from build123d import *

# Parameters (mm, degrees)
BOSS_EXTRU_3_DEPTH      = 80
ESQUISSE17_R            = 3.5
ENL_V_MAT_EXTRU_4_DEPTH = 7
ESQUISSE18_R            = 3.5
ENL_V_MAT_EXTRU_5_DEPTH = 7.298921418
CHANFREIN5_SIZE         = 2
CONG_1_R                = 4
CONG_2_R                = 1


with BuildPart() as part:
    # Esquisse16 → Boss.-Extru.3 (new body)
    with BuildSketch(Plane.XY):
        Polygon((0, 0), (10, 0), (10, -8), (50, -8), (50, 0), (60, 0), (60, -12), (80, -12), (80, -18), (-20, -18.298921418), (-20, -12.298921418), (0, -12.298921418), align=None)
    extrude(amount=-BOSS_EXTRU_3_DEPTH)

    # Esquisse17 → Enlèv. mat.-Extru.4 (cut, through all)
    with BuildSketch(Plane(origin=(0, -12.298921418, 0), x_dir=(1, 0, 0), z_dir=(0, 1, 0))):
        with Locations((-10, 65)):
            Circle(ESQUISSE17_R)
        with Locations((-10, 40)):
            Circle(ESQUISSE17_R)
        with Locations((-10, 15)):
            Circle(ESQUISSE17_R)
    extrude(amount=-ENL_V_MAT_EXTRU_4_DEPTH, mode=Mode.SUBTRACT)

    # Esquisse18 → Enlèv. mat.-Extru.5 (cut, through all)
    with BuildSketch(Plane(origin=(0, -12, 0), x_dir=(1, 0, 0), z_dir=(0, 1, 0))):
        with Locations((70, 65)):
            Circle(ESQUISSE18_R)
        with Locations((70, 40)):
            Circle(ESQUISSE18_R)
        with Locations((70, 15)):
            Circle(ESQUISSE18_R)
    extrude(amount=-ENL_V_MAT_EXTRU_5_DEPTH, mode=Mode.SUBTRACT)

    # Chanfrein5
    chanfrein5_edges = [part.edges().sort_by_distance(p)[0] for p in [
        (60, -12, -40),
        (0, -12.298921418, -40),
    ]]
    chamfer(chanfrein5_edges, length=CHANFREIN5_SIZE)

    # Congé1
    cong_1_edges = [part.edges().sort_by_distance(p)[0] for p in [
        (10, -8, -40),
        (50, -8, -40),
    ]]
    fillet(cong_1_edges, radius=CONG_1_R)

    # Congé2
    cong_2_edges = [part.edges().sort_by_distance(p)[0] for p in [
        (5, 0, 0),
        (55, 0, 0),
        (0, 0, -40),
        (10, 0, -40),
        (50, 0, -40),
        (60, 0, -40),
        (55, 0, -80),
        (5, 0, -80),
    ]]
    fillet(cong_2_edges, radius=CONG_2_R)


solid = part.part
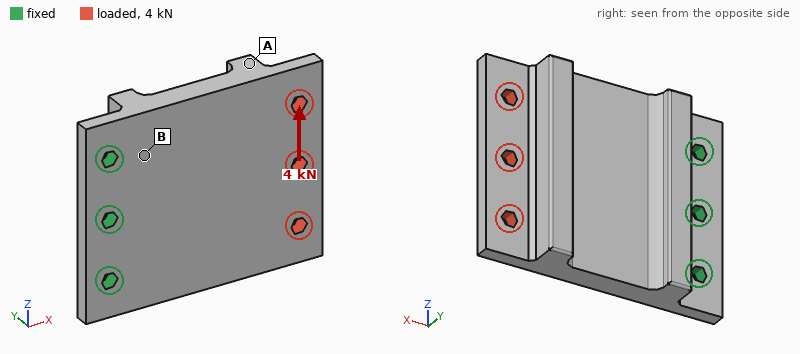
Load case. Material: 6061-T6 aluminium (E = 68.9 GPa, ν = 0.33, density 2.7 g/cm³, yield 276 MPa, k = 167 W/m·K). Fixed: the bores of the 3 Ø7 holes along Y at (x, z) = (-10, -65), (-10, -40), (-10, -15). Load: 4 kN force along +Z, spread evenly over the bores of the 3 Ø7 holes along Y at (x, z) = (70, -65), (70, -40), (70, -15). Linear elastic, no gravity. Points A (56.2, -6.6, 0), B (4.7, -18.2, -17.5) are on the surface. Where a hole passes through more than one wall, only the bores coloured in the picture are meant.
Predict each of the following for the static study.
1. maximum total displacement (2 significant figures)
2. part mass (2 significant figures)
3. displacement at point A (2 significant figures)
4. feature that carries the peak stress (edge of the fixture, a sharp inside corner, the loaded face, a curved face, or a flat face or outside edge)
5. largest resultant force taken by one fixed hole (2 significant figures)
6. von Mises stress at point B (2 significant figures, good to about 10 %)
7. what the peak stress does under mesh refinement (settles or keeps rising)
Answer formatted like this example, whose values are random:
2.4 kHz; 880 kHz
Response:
100 µm; 220 g; 71 µm; edge of the fixture; 6.0 kN; 37 MPa; keeps rising
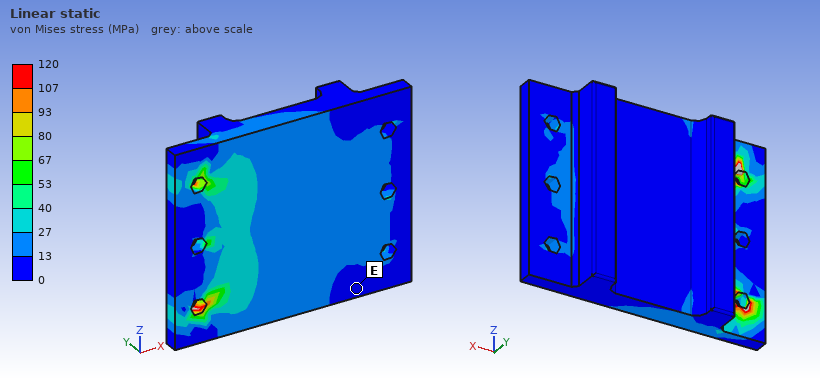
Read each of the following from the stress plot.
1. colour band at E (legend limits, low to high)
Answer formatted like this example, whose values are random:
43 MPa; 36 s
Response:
0 to 13 MPa
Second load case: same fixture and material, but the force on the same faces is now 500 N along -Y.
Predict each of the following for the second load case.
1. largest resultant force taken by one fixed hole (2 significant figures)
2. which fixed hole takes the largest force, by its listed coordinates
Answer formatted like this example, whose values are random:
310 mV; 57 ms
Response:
250 N; (-10, -40)
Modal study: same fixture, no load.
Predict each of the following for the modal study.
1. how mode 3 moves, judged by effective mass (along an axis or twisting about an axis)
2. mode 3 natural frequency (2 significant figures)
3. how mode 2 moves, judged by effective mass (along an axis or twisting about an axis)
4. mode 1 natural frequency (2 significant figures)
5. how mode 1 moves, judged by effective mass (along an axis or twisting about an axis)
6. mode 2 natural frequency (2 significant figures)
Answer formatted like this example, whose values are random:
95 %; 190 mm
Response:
along Z; 4500 Hz; twisting about X; 740 Hz; along Y; 2500 Hz
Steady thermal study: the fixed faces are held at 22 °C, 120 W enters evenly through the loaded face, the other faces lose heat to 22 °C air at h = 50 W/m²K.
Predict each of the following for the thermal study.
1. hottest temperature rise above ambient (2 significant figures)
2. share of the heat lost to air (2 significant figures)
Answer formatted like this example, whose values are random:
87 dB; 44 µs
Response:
74 K; 28 %
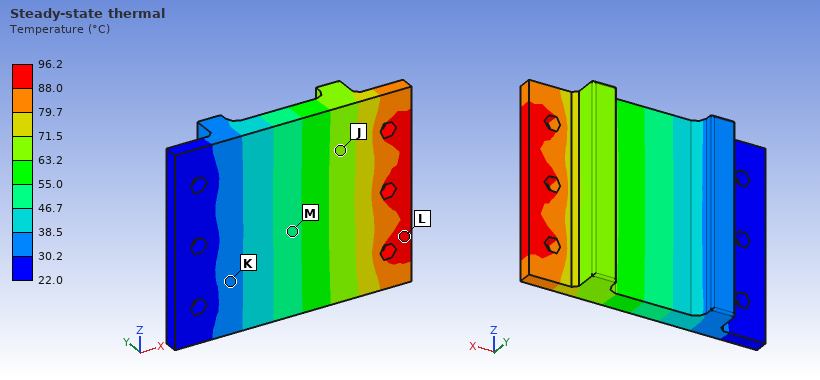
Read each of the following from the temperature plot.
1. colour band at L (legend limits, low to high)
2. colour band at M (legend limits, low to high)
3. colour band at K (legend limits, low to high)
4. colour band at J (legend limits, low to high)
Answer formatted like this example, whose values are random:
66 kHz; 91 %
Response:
88.0 to 96.2 °C; 46.7 to 55.0 °C; 30.2 to 38.5 °C; 63.2 to 71.5 °C
